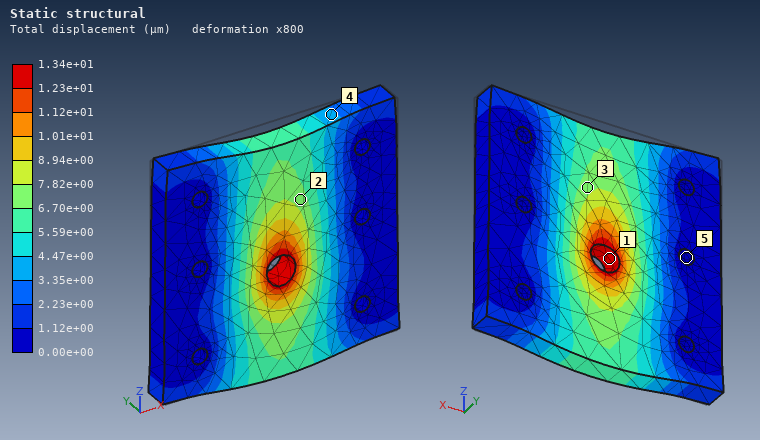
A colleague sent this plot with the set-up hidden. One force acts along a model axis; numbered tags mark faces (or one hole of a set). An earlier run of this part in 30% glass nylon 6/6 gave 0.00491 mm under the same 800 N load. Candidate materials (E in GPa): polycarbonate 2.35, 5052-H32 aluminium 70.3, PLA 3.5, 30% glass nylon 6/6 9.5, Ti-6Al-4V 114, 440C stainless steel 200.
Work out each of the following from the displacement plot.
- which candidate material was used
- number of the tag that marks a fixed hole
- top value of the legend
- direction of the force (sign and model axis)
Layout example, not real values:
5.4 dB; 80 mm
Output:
PLA; 5; 1.34e+01 µm; -Z
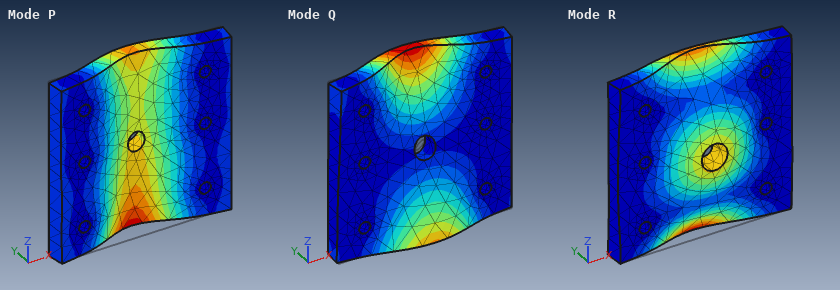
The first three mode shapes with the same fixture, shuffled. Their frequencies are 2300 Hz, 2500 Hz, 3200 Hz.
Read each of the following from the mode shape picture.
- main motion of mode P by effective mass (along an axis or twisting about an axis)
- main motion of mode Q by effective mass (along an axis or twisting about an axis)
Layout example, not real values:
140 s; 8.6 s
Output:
along Y; twisting about X
